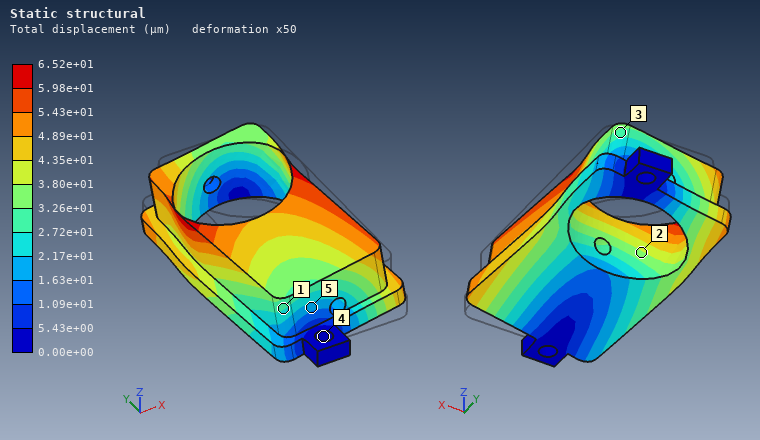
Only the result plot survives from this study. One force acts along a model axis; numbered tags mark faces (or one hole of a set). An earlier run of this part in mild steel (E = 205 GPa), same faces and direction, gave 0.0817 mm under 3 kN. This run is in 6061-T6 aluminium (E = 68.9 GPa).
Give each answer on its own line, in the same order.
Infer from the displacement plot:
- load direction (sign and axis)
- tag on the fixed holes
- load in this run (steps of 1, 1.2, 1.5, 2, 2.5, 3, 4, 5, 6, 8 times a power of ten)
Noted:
-X
4
800 N
